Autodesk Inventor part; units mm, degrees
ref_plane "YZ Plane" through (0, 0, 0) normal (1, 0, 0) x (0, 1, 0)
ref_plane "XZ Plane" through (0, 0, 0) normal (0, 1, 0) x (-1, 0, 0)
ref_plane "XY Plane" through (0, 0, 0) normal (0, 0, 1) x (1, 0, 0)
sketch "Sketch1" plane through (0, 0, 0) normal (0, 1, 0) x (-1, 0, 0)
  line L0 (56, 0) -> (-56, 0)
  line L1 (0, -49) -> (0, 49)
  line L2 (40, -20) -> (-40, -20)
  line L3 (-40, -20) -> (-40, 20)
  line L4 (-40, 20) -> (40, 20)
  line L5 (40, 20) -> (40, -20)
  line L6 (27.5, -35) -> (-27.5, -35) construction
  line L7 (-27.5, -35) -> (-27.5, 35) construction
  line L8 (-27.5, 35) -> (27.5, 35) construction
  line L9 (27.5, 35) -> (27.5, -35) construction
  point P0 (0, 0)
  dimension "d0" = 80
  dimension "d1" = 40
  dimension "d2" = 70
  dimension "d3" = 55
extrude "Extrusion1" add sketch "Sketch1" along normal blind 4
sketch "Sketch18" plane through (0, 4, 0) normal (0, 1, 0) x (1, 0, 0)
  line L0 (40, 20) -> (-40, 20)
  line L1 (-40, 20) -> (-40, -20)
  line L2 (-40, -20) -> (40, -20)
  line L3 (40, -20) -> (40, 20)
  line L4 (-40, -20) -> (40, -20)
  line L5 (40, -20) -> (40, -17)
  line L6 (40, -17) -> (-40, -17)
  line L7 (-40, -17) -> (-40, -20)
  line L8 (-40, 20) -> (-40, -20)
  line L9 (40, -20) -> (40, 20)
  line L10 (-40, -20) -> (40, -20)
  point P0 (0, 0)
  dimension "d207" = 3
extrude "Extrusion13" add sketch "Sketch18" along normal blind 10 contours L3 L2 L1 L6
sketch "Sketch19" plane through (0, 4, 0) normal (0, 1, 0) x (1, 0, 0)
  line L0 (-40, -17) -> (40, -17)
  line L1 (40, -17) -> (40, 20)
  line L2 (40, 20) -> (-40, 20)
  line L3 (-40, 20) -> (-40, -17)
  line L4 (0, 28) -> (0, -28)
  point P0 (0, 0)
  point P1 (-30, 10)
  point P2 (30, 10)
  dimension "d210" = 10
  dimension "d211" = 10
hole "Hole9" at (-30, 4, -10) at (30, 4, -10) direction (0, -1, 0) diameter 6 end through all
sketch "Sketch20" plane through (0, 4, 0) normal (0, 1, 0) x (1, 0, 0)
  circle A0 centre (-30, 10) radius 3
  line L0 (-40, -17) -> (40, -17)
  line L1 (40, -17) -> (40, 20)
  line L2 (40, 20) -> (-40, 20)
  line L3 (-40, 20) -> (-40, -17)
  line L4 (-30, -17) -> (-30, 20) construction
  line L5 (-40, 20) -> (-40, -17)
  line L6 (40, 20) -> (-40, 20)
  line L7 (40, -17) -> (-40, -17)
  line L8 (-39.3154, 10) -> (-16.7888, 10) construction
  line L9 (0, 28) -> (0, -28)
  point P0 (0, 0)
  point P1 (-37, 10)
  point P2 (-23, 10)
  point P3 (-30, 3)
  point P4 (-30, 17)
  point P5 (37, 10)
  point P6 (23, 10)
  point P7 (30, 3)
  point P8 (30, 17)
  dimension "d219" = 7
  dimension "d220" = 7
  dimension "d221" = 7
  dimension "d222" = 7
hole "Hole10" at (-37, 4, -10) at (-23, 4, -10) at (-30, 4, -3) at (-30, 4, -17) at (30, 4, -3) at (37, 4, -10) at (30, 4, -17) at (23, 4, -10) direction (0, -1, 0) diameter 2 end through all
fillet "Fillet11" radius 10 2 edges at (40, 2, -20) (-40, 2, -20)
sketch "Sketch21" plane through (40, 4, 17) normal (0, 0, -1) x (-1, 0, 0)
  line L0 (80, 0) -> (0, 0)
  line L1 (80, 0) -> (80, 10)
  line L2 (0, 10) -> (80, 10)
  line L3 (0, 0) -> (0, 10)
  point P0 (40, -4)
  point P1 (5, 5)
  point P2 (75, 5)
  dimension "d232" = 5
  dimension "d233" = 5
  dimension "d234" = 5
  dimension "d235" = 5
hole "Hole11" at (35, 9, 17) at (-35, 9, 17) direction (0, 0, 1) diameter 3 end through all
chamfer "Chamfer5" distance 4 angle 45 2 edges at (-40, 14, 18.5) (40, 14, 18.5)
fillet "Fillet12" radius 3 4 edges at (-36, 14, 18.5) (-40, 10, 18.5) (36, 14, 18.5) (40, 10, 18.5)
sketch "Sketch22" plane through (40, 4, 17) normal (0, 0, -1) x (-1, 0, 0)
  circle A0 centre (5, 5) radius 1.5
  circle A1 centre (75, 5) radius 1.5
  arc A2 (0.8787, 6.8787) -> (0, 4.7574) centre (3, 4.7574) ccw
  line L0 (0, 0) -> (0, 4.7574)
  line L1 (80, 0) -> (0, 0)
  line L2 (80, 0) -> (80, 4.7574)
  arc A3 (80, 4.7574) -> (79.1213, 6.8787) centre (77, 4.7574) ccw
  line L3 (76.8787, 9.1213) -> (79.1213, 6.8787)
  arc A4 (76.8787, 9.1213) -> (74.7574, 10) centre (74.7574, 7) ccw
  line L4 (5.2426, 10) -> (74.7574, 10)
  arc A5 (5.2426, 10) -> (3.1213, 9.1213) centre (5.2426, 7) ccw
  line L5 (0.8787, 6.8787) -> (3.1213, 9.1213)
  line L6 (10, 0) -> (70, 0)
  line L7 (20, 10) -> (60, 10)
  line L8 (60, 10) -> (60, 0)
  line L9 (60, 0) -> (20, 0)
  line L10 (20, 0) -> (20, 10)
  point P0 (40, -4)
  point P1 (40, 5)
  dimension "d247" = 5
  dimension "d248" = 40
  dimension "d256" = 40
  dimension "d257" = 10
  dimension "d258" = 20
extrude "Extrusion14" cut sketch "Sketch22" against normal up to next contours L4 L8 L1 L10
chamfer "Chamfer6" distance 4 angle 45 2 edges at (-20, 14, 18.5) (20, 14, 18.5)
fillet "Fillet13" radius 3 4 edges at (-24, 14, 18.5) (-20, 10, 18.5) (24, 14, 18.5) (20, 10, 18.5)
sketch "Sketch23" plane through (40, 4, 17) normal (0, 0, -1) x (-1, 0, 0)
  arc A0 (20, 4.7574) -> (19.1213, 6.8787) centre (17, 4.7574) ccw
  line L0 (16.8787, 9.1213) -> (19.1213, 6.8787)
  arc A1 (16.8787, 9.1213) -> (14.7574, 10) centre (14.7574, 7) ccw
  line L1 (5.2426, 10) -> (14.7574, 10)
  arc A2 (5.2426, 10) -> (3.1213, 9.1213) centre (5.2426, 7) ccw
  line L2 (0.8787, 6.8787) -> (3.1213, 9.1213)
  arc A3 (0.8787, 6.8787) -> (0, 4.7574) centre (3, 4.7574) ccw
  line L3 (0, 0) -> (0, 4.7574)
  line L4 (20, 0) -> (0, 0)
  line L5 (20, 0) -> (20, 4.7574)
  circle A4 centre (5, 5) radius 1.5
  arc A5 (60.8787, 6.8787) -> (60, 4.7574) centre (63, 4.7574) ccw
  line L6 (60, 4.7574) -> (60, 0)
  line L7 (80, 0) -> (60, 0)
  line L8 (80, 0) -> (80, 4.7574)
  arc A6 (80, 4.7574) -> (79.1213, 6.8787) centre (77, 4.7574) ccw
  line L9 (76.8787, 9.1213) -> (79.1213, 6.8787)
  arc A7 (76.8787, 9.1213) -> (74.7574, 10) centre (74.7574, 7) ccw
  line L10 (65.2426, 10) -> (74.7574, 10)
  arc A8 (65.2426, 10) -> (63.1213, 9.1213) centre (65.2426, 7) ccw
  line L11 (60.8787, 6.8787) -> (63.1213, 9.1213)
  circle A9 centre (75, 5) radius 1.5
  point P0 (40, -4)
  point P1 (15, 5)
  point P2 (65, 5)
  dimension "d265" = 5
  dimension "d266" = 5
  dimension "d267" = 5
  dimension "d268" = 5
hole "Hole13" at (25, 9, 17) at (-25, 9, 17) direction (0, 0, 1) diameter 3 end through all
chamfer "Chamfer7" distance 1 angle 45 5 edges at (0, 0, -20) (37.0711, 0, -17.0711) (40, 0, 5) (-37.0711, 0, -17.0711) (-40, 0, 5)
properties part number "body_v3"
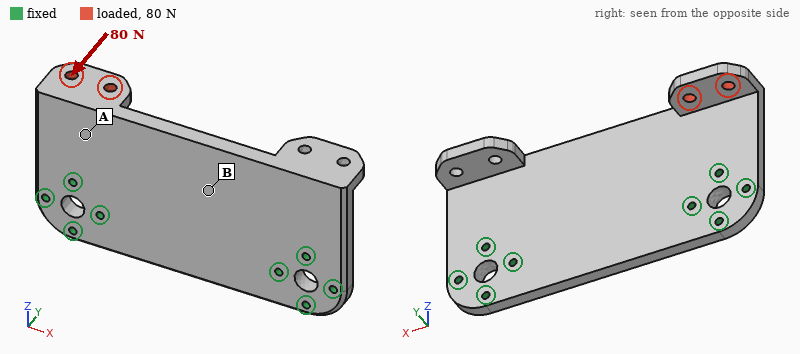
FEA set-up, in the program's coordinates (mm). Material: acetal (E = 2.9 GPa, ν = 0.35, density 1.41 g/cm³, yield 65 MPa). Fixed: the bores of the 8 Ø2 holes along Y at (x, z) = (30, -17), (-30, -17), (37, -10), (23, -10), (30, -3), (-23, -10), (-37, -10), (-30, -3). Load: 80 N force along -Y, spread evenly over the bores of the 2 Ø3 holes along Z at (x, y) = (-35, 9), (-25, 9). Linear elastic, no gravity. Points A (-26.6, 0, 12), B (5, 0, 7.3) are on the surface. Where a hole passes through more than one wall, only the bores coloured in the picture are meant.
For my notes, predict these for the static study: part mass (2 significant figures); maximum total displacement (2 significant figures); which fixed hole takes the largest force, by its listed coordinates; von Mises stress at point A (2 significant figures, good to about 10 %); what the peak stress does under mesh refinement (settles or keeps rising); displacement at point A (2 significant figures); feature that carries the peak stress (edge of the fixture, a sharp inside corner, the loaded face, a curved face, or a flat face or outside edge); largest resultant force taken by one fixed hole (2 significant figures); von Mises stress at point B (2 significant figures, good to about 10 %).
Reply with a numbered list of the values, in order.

1. 19 g
2. 0.92 mm
3. (-30, -3)
4. 7.1 MPa
5. keeps rising
6. 0.39 mm
7. edge of the fixture
8. 150 N
9. 3.3 MPa
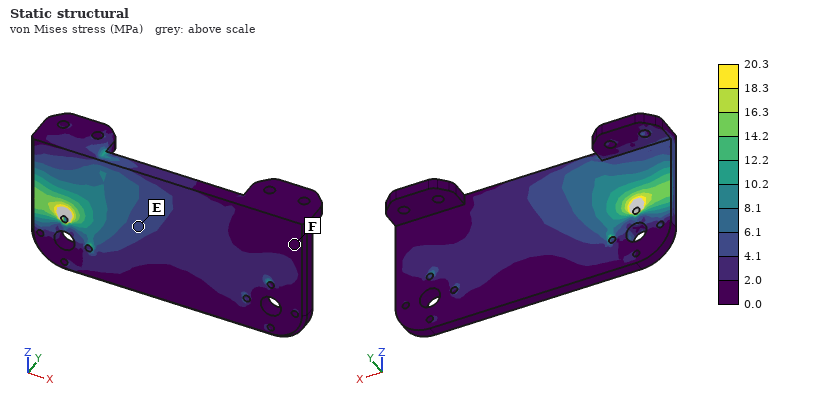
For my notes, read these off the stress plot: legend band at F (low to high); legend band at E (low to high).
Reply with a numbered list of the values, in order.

1. 0.0 to 2.0 MPa
2. 4.1 to 6.1 MPa
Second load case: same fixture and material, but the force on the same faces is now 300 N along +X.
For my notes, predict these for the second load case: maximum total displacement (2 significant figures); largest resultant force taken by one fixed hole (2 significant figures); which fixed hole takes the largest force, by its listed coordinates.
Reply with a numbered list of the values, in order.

1. 1.00 mm
2. 140 N
3. (-30, -3)
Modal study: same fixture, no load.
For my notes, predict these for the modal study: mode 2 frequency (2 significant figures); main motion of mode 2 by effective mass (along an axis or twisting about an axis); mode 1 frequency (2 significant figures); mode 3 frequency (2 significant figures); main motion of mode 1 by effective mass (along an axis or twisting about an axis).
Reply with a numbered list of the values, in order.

1. 1400 Hz
2. twisting about Z
3. 960 Hz
4. 1700 Hz
5. along Y
